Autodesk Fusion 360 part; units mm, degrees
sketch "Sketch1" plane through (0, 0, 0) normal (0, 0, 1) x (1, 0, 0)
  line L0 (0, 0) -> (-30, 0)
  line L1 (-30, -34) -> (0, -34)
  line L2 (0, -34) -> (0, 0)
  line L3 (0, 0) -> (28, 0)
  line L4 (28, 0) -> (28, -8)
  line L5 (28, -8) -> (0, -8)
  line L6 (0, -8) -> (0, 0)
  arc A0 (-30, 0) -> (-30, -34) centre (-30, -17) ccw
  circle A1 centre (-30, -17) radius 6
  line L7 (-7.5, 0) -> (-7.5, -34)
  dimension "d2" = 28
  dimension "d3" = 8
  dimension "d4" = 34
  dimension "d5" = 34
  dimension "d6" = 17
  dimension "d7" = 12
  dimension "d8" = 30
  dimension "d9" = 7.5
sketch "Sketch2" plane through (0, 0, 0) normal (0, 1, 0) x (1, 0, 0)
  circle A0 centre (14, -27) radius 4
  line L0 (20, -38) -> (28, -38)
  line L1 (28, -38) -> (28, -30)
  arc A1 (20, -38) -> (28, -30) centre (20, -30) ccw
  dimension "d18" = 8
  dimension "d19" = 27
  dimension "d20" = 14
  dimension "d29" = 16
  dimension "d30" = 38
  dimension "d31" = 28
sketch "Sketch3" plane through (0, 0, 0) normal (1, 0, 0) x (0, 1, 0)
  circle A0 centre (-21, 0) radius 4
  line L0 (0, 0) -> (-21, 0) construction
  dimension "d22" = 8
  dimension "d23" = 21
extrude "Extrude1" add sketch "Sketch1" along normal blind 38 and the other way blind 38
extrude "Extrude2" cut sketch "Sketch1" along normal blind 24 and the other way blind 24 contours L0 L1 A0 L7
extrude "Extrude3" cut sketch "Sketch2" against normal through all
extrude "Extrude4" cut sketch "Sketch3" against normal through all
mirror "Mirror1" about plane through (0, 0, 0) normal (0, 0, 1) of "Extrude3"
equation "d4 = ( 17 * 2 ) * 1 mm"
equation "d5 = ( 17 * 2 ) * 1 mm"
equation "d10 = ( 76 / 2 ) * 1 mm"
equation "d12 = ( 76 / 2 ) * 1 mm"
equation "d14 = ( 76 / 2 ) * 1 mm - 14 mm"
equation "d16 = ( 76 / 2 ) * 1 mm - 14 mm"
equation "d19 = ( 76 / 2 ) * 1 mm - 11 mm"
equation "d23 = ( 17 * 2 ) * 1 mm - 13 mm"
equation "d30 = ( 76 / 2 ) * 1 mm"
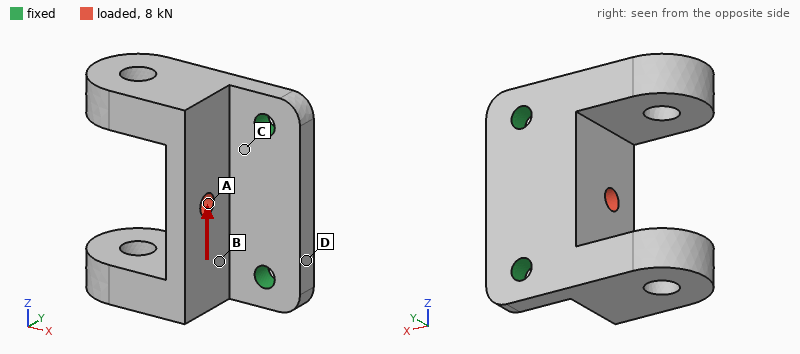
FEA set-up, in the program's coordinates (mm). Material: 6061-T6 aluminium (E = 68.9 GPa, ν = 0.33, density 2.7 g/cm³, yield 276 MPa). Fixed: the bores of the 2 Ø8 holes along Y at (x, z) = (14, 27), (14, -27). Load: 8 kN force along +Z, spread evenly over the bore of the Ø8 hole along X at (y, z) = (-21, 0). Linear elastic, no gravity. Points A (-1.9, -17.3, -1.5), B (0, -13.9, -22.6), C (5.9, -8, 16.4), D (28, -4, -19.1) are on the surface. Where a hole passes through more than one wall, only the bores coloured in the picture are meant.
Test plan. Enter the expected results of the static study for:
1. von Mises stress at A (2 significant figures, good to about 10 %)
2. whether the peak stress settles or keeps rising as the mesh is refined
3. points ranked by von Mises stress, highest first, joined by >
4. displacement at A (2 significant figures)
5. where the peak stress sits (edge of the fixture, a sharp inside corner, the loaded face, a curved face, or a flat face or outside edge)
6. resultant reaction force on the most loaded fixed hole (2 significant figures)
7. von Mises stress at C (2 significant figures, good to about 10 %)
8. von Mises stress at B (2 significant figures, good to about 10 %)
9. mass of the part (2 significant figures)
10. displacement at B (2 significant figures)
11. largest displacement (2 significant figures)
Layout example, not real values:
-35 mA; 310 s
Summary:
84 MPa; keeps rising; A > C > B > D; 0.036 mm; edge of the fixture; 5.2 kN; 53 MPa; 38 MPa; 180 g; 0.034 mm; 0.11 mm
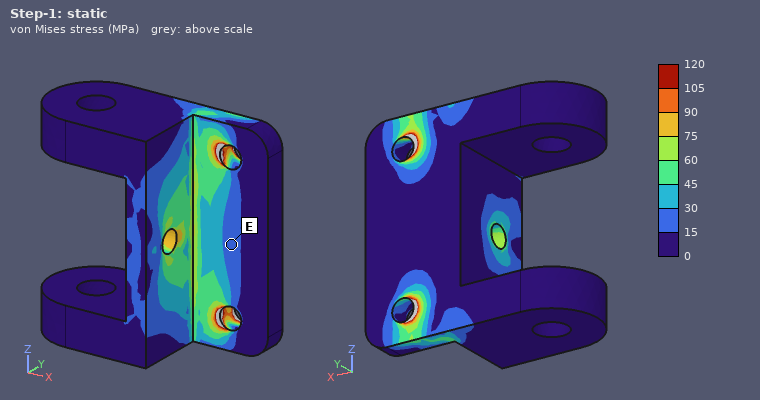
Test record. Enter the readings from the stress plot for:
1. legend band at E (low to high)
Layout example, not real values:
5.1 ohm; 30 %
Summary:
15 to 30 MPa
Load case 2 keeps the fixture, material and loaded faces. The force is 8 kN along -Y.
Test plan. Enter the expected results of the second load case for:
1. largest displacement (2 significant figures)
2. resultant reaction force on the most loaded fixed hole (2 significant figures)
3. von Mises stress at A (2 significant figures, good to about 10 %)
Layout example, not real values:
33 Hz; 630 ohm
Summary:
0.36 mm; 4.1 kN; 42 MPa
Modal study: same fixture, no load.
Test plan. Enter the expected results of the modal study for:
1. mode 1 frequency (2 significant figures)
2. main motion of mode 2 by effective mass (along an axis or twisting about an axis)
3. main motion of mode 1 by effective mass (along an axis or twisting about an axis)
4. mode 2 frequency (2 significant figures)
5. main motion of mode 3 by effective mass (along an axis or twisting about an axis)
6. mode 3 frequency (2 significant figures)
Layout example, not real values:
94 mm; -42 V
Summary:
1500 Hz; twisting about X; along Y; 2000 Hz; along Z; 3700 Hz
